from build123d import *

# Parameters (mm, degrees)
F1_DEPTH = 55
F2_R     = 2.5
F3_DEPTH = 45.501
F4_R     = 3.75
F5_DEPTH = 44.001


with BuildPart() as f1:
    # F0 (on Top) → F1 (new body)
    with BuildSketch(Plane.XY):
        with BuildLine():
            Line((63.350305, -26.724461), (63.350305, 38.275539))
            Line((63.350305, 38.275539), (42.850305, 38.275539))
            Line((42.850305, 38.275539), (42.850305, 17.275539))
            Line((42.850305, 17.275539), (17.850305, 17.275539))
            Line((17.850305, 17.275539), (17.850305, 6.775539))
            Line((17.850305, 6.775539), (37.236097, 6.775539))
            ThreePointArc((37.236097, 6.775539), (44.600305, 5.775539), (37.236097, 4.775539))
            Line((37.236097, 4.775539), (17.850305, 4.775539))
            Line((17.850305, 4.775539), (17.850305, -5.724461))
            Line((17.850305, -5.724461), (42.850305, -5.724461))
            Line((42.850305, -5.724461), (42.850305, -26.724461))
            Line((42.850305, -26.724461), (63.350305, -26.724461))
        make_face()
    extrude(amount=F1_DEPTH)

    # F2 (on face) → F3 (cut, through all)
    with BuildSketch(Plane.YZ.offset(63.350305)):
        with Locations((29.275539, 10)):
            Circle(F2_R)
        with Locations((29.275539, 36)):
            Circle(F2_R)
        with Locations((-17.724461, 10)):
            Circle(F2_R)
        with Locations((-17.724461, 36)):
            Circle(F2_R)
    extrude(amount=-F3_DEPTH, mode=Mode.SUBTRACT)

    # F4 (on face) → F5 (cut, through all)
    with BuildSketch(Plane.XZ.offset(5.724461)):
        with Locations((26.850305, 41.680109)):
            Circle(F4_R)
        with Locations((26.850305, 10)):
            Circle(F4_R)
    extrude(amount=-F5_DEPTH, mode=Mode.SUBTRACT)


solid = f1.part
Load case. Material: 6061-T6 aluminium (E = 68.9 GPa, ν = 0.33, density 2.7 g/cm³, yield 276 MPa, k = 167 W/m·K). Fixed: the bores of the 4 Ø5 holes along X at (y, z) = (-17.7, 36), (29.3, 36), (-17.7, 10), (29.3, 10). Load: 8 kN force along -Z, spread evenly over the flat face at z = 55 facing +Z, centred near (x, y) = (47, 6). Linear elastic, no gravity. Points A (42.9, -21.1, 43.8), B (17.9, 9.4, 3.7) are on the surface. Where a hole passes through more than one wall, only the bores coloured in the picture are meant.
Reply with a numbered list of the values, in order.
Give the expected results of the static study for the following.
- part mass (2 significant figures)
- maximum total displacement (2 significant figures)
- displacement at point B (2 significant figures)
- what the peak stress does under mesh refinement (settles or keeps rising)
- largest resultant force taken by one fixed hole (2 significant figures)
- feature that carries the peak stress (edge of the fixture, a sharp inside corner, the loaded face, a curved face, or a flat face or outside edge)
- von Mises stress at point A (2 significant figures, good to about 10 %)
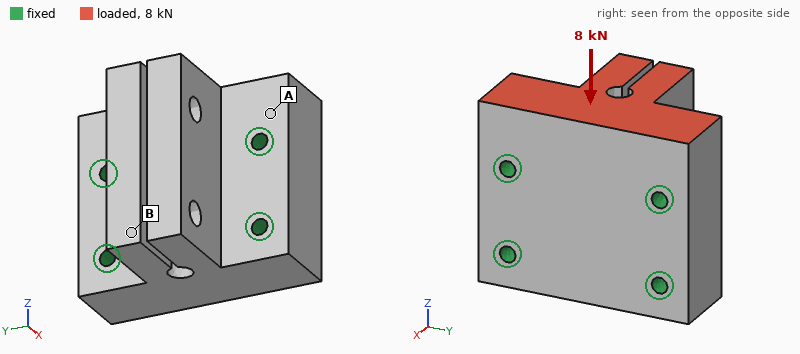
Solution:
1. 260 g
2. 9.8 µm
3. 6.9 µm
4. keeps rising
5. 2.9 kN
6. edge of the fixture
7. 6.9 MPa
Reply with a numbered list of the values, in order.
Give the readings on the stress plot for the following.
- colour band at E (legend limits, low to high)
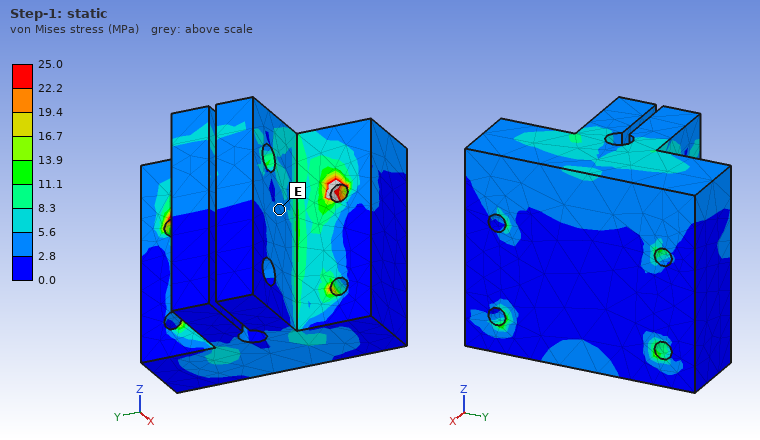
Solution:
1. 2.8 to 5.6 MPa
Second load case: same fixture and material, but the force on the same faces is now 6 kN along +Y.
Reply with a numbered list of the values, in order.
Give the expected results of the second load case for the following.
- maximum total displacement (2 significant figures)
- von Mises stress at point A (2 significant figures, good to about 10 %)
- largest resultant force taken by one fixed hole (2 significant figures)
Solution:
1. 40 µm
2. 4.8 MPa
3. 3.5 kN
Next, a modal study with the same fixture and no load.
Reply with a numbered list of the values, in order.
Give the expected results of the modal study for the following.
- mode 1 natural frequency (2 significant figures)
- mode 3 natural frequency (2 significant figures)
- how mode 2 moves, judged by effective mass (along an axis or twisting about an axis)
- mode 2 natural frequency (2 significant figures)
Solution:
1. 7400 Hz
2. 11 kHz
3. along Y
4. 7800 Hz
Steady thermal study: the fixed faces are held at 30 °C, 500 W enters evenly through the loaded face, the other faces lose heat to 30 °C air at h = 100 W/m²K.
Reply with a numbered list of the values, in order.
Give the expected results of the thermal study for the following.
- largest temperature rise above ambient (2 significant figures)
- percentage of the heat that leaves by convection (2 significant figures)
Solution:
1. 62 K
2. 6.4 %
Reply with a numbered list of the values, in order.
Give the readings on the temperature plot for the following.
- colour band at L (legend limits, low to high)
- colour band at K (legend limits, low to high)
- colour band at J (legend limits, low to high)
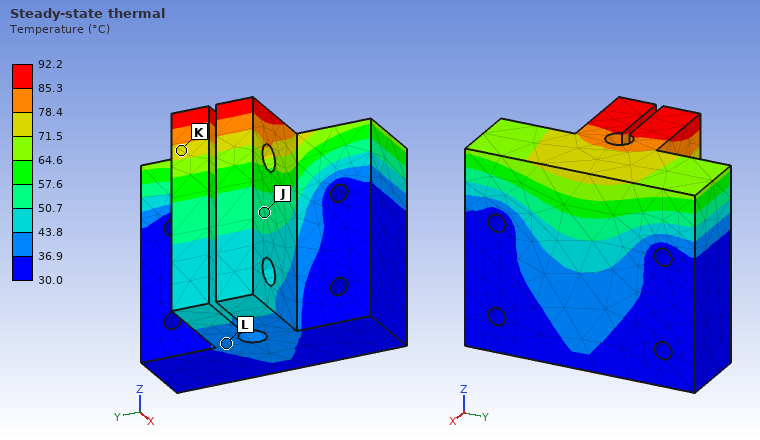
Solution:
1. 36.9 to 43.8 °C
2. 71.5 to 78.4 °C
3. 50.7 to 57.6 °C
